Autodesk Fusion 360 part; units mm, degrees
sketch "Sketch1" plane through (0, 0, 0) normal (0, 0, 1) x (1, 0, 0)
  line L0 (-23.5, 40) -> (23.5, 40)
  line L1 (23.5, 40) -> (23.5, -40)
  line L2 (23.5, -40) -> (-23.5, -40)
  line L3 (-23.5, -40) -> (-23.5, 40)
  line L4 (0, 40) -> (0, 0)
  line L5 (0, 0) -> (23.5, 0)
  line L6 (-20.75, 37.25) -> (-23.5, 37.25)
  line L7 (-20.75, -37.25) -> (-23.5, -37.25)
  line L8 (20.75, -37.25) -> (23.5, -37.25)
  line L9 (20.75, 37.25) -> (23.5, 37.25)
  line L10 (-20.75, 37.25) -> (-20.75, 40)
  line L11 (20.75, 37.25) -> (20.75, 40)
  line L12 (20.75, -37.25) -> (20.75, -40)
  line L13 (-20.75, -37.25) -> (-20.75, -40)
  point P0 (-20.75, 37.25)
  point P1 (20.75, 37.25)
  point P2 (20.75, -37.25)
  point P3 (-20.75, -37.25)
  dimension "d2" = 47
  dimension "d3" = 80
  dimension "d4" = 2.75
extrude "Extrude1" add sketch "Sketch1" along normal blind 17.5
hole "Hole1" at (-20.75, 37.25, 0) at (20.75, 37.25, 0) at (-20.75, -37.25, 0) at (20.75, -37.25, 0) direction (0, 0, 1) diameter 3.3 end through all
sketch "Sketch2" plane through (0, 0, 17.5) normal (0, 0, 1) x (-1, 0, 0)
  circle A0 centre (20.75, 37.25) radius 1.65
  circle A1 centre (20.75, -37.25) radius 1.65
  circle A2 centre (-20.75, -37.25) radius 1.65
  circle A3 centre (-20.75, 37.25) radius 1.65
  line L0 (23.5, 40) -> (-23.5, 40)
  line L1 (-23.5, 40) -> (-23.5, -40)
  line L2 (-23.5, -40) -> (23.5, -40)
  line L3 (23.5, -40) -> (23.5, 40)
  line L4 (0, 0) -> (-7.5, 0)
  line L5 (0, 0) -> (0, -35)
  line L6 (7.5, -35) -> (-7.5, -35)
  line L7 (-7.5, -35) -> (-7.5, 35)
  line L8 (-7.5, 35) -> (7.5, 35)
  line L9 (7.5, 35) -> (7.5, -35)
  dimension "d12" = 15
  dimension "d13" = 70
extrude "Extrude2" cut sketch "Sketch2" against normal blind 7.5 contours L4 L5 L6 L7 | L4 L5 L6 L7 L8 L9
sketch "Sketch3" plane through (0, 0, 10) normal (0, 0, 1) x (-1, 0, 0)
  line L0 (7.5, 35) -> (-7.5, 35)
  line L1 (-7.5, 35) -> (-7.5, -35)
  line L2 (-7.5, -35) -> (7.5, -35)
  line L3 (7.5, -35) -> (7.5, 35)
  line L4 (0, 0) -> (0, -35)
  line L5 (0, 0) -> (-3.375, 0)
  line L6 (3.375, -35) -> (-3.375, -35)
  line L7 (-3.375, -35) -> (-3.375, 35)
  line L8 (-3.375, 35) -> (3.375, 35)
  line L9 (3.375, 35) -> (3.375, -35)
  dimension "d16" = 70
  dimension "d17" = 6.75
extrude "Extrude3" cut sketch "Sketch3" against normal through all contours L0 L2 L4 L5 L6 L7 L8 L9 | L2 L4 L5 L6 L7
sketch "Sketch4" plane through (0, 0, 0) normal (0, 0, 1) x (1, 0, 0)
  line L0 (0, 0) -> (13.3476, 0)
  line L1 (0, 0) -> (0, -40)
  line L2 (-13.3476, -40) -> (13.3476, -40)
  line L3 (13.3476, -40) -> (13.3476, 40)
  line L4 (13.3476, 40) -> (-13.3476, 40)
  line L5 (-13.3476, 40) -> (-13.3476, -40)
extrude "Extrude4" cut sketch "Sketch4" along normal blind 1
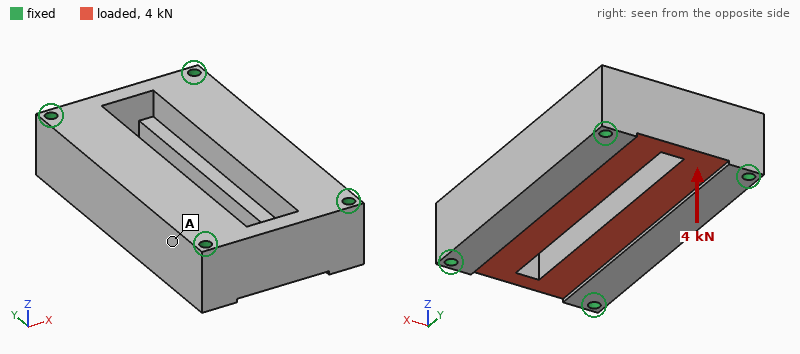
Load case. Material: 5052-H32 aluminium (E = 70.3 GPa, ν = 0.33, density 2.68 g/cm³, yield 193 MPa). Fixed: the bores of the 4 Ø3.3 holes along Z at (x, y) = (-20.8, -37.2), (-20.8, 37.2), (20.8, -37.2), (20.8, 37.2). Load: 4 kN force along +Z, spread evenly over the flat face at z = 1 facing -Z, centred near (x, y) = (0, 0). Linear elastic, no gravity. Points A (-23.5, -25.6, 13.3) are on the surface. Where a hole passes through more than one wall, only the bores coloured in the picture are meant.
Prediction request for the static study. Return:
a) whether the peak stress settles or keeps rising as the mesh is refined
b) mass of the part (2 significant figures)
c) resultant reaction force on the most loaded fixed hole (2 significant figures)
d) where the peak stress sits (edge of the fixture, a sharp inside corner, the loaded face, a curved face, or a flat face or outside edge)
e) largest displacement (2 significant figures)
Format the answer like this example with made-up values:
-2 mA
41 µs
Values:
keeps rising
140 g
1.0 kN
edge of the fixture
16 µm
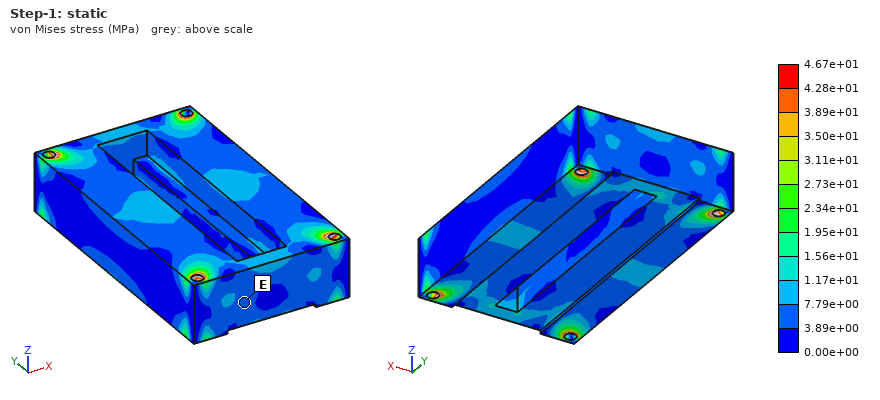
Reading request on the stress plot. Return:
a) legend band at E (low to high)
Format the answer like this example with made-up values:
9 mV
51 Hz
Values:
3.89e+00 to 7.79e+00 MPa
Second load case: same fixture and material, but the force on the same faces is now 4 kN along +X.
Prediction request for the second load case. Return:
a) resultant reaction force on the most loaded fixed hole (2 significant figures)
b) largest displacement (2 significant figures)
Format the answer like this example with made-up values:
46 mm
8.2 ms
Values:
1.2 kN
12 µm
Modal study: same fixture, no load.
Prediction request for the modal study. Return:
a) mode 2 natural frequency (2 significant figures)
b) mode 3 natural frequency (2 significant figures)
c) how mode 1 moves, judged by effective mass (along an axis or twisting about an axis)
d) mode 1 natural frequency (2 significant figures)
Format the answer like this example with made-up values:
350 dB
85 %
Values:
10 kHz
10 kHz
along Z
9800 Hz
